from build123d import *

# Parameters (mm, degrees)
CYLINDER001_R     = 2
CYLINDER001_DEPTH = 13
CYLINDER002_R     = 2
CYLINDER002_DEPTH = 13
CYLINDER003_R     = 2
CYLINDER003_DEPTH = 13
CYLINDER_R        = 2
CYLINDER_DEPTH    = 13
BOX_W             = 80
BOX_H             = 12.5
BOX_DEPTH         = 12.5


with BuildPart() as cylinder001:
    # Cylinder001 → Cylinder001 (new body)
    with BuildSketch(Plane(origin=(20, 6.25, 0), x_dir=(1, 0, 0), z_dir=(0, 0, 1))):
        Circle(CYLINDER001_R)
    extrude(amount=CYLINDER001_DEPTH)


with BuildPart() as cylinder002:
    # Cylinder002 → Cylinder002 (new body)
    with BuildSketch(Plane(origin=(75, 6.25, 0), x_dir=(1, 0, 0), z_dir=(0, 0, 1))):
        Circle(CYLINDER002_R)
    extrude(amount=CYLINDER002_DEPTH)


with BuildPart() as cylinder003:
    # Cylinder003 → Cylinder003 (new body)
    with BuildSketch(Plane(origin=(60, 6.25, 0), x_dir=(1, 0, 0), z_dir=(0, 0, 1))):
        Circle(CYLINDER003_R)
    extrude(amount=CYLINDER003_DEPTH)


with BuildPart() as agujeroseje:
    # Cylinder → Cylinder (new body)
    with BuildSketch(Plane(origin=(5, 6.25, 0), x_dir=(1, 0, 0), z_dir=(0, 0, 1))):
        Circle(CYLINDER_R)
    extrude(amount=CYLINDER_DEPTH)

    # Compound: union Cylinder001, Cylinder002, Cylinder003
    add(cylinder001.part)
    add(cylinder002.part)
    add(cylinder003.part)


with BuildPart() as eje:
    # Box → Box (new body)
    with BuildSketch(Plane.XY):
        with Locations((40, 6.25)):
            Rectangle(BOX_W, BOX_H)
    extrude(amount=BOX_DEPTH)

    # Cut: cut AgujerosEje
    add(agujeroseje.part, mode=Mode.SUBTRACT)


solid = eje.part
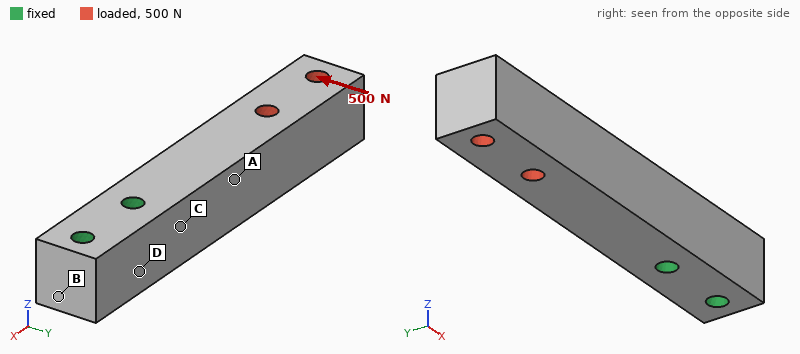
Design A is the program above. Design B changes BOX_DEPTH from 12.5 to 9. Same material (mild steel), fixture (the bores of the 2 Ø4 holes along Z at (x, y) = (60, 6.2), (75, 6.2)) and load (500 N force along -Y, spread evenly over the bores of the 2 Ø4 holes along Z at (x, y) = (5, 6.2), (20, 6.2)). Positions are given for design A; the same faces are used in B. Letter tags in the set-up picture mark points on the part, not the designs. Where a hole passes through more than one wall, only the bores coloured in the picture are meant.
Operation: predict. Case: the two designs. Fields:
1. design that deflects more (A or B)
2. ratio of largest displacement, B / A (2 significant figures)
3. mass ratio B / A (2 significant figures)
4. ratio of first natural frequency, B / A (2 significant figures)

B
1.4
0.72
0.81
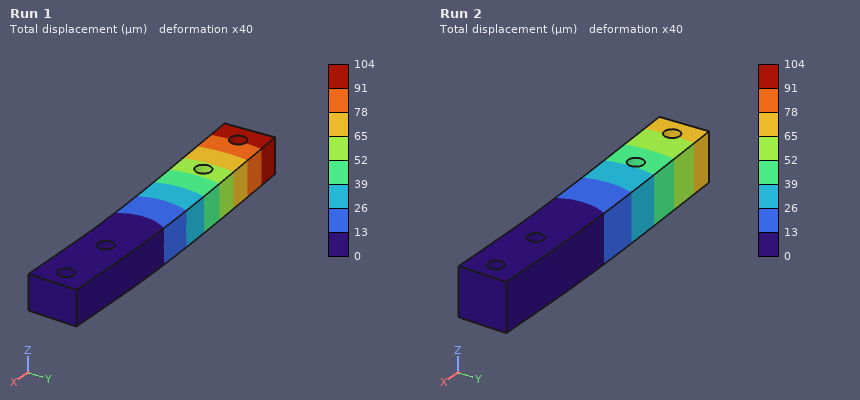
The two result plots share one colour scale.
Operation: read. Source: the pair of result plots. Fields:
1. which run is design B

Run 1
